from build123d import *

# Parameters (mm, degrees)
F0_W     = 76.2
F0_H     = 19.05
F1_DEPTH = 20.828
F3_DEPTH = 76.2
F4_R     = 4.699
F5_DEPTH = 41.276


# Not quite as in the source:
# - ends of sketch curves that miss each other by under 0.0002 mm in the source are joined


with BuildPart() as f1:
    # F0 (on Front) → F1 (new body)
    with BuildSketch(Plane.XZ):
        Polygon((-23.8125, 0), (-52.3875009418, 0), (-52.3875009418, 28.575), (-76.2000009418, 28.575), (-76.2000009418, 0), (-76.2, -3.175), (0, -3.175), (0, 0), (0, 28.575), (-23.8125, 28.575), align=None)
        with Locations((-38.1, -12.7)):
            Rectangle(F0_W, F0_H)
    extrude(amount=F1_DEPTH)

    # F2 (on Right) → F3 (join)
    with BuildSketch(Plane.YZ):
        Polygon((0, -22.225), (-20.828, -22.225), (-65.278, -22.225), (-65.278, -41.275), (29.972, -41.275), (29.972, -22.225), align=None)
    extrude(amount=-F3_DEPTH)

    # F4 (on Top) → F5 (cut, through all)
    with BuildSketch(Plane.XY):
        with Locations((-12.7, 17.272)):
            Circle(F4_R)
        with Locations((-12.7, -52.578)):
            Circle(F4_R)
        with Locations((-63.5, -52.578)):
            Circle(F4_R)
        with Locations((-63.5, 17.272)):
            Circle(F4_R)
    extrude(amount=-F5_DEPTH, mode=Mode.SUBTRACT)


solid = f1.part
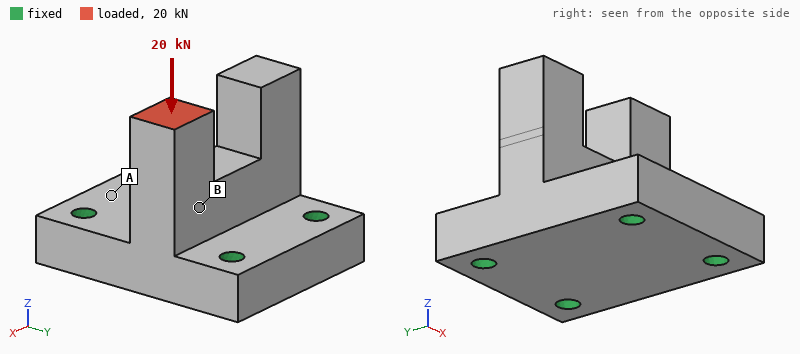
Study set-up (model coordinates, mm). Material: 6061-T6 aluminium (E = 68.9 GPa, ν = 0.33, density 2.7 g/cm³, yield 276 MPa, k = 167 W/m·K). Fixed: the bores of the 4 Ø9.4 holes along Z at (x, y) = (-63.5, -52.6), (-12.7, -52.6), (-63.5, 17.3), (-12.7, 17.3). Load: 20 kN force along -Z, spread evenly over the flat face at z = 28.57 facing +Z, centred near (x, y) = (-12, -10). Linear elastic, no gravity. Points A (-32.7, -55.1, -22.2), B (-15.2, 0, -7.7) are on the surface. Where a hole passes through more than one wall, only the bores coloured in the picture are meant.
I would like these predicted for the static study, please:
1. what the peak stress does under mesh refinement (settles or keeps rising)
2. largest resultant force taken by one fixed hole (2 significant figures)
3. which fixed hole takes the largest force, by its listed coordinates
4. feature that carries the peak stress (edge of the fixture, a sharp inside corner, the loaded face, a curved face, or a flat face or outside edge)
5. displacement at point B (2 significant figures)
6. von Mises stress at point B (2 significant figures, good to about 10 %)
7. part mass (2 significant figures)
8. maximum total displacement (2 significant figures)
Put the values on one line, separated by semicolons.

keeps rising; 12 kN; (-12.7, 17.3); edge of the fixture; 38 µm; 37 MPa; 530 g; 96 µm
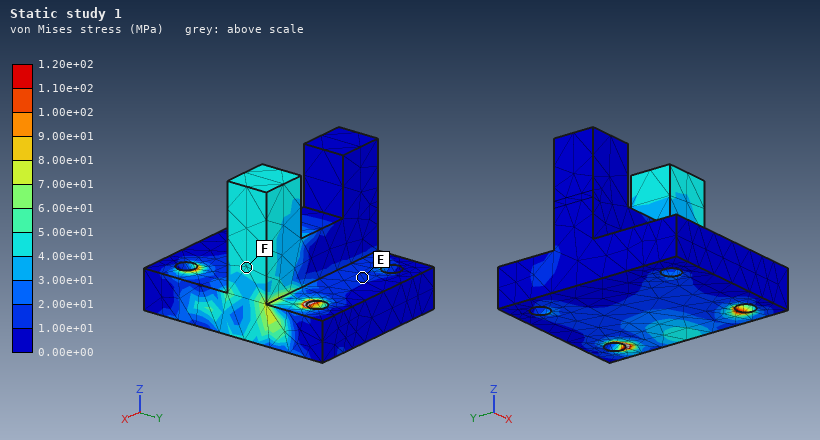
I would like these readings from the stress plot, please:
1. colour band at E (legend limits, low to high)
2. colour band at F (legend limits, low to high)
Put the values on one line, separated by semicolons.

1.00e+01 to 2.00e+01 MPa; 4.00e+01 to 5.00e+01 MPa
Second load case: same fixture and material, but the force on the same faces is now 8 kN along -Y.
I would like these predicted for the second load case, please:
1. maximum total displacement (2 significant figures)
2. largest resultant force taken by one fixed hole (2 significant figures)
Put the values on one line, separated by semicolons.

0.36 mm; 7.2 kN
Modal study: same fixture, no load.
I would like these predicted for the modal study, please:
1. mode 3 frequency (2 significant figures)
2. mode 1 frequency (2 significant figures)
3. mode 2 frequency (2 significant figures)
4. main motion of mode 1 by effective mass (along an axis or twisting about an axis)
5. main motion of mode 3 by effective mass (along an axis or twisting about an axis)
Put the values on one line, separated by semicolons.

6200 Hz; 5100 Hz; 5800 Hz; along Y; along X
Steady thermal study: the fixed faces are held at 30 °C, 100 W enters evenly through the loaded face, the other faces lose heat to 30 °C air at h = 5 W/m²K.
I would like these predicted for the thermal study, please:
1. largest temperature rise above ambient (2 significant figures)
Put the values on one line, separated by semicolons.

64 K
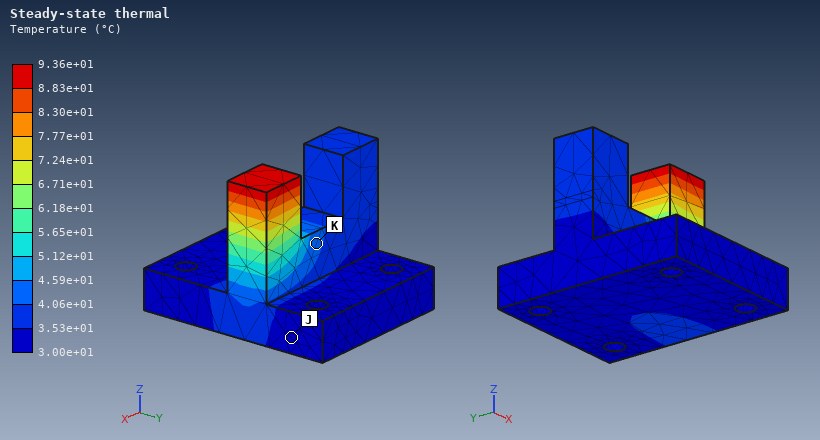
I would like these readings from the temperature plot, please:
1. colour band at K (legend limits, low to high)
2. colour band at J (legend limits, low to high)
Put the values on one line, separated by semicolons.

4.06e+01 to 4.59e+01 °C; 3.00e+01 to 3.53e+01 °C
